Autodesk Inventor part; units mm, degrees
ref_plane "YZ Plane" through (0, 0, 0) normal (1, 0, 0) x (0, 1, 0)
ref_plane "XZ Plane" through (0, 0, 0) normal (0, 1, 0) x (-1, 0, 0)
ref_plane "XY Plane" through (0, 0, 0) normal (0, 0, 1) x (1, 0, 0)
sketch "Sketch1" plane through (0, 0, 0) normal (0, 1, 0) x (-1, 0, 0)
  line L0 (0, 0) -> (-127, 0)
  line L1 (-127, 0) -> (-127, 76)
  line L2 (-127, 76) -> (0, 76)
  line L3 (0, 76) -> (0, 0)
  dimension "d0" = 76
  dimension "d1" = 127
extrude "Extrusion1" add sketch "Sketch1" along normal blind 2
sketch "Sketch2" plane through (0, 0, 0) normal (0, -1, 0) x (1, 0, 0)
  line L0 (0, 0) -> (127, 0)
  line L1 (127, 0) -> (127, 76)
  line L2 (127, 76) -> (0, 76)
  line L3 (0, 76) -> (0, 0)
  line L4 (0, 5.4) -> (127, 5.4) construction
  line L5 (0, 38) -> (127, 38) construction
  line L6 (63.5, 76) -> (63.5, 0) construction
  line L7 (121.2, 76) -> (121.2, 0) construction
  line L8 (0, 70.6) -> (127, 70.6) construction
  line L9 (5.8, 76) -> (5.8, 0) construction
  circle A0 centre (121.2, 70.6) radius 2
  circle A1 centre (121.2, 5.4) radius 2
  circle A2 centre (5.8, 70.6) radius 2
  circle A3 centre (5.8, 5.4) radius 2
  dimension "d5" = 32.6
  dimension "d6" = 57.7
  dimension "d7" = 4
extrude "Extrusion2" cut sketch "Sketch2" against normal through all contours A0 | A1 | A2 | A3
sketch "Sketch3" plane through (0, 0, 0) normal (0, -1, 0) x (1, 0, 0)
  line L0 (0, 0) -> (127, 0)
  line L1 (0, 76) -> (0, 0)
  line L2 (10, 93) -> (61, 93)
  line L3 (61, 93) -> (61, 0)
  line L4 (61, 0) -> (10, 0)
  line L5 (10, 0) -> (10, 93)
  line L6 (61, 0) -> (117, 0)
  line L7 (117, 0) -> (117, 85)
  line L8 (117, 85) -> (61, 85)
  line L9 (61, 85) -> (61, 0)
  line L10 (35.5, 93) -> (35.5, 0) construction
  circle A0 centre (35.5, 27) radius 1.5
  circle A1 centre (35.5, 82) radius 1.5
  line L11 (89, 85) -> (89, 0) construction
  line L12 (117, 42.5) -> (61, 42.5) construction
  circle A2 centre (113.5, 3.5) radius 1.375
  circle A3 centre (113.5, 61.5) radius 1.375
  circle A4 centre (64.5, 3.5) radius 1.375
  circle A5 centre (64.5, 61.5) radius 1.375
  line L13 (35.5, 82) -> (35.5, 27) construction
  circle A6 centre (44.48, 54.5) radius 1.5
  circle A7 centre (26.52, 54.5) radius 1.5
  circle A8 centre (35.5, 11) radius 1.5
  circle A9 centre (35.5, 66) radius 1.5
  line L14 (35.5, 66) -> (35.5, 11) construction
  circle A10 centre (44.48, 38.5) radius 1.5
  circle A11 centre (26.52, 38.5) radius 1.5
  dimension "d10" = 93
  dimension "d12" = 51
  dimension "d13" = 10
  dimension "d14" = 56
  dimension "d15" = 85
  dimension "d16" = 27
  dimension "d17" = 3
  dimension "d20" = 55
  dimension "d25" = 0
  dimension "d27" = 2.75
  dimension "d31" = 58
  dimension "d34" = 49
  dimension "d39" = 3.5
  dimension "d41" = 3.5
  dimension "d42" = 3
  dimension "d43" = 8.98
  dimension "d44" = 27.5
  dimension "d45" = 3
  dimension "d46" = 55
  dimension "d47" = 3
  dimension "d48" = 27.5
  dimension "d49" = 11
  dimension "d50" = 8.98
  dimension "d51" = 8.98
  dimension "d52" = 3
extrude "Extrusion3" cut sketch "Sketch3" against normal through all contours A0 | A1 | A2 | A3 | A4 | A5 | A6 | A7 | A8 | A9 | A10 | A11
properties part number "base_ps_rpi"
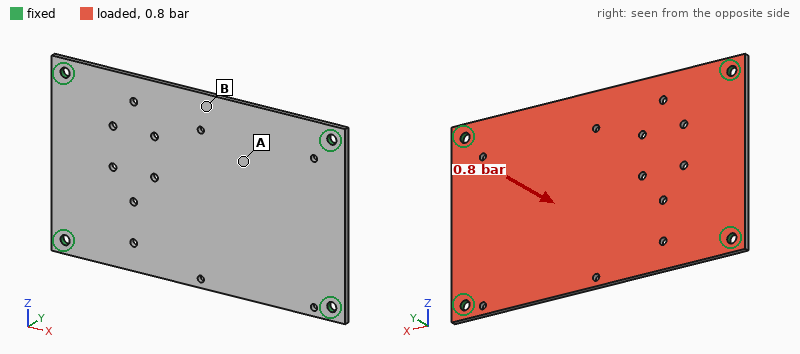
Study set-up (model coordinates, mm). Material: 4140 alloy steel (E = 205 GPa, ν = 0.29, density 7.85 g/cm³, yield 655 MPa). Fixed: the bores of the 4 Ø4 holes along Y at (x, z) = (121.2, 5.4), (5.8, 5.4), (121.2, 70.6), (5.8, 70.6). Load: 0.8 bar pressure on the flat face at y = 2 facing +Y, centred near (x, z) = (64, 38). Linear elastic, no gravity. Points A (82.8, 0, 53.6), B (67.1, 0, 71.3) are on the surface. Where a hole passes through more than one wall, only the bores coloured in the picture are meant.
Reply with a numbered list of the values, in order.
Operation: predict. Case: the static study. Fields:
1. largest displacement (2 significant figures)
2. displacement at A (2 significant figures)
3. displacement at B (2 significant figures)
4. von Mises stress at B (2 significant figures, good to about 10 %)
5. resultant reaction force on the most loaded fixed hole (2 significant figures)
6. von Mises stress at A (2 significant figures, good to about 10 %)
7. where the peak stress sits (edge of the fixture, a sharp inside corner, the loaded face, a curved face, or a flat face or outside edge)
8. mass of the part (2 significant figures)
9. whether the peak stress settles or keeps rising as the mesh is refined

1. 0.38 mm
2. 0.31 mm
3. 0.36 mm
4. 84 MPa
5. 190 N
6. 52 MPa
7. edge of the fixture
8. 150 g
9. keeps rising
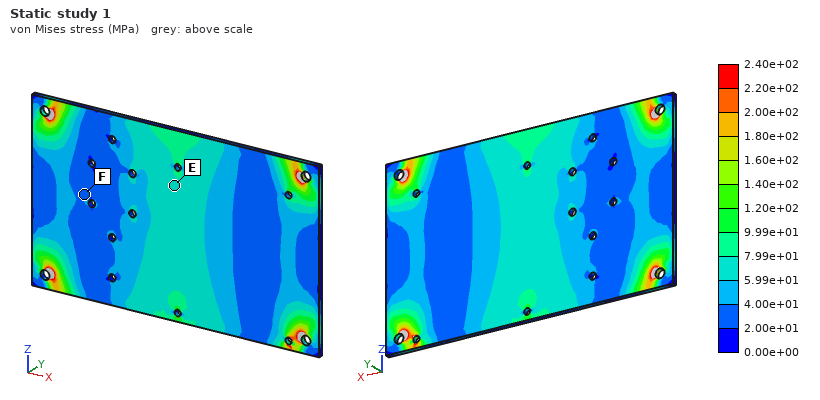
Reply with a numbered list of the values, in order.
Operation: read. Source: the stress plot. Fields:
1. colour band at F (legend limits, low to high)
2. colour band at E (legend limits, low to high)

1. 2.00e+01 to 4.00e+01 MPa
2. 5.99e+01 to 7.99e+01 MPa
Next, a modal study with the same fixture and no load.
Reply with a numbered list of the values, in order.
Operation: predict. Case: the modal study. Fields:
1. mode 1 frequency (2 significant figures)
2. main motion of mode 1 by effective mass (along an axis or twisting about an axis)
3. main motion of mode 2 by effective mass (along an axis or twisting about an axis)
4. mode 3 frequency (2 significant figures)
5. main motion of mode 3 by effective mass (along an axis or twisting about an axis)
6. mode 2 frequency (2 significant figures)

1. 670 Hz
2. along Y
3. twisting about X
4. 1800 Hz
5. twisting about Z
6. 1100 Hz
